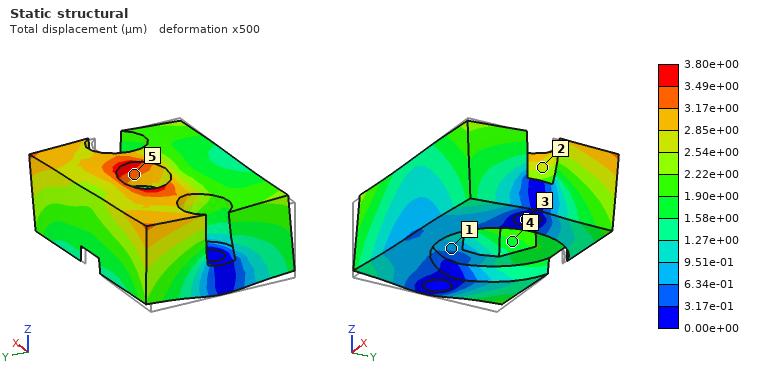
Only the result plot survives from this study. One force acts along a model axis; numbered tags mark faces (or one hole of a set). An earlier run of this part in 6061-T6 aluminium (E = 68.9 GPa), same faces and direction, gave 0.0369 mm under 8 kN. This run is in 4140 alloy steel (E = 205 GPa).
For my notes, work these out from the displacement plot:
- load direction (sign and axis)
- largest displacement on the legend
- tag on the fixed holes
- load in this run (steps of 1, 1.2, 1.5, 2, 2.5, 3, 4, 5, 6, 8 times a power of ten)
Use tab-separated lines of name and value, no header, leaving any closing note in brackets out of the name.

load direction	+X
largest displacement on the legend	3.80e+00 µm
tag on the fixed holes	3
load in this run	2.5 kN
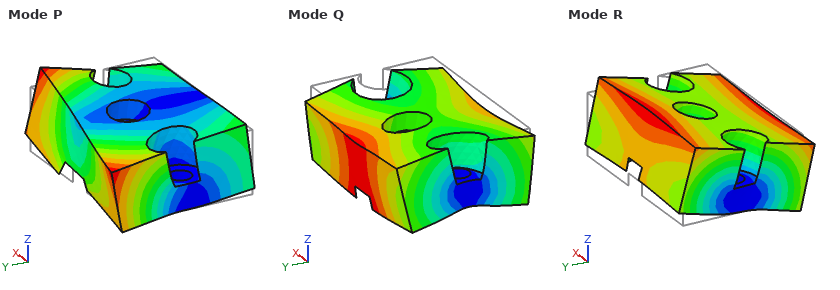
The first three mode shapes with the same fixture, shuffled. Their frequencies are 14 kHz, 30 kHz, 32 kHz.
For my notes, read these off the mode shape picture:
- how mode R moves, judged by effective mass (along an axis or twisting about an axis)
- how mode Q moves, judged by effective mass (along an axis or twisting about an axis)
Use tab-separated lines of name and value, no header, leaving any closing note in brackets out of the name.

how mode R moves, judged by effective mass	along Y
how mode Q moves, judged by effective mass	along Z
